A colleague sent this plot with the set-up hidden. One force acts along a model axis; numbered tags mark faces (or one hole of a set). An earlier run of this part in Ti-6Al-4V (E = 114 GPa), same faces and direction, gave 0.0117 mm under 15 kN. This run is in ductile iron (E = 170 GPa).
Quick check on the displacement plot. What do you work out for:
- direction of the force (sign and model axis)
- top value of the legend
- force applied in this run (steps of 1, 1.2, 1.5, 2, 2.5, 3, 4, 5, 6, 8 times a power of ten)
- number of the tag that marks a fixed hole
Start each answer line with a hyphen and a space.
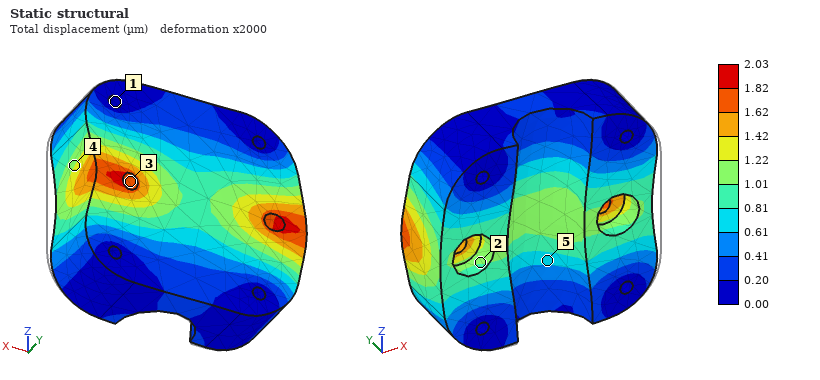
- -X
- 2.03 µm
- 4 kN
- 1
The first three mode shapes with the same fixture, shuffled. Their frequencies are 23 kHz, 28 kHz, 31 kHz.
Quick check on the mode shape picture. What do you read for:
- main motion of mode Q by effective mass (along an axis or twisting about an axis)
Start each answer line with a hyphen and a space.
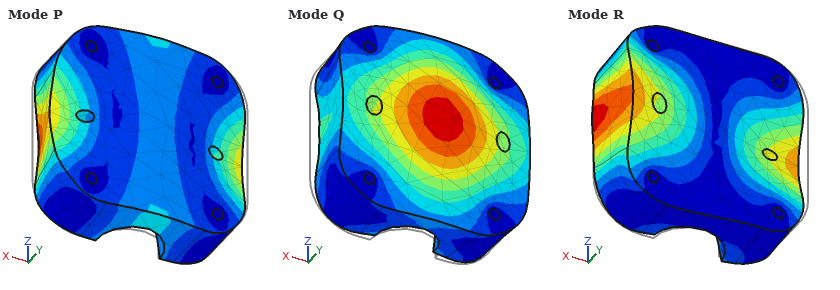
- along Y
